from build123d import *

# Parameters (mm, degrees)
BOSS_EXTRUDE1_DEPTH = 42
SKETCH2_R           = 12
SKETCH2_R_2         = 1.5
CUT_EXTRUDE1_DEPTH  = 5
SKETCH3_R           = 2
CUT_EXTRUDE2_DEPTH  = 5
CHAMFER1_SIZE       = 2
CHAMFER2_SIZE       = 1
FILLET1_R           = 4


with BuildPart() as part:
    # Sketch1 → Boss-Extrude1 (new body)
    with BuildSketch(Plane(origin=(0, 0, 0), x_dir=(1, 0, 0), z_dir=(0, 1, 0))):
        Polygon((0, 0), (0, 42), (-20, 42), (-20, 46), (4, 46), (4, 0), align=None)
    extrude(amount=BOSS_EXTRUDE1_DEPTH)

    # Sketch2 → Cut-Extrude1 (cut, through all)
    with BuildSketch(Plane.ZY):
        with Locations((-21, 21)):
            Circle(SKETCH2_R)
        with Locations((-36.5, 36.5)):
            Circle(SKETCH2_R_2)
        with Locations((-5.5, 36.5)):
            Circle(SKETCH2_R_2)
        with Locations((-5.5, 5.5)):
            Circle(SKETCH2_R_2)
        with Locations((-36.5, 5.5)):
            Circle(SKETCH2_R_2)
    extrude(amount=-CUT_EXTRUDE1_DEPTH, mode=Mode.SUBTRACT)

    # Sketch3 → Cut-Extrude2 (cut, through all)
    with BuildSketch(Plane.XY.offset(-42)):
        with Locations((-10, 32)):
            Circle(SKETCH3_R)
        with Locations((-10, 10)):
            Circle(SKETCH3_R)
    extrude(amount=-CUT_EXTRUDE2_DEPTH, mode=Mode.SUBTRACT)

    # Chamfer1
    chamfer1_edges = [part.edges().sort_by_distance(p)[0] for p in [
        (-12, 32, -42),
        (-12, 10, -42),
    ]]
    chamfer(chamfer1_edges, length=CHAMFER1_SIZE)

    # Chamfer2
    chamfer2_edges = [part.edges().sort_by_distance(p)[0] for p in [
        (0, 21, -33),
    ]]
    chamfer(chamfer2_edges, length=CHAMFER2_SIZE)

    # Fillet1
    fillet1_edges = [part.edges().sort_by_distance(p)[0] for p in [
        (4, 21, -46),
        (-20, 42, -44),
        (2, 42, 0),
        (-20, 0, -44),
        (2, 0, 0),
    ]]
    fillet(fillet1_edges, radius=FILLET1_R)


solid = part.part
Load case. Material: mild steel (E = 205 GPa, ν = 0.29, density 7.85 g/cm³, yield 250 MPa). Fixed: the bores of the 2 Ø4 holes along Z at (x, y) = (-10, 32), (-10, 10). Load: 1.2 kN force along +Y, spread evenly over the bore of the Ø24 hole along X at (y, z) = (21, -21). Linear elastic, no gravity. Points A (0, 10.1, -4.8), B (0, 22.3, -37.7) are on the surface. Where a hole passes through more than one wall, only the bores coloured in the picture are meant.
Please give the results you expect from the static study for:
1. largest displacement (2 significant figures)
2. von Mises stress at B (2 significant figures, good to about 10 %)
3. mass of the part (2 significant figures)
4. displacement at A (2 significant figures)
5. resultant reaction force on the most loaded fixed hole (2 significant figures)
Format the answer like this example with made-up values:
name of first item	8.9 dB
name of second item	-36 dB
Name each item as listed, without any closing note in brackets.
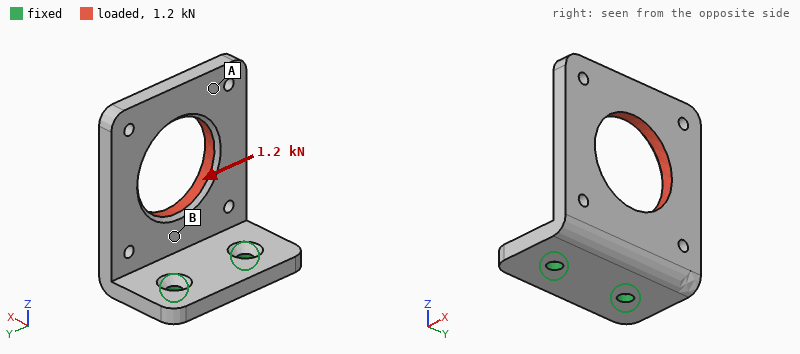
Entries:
largest displacement	0.11 mm
von Mises stress at B	95 MPa
mass of the part	69 g
displacement at A	0.094 mm
resultant reaction force on the most loaded fixed hole	1.4 kN
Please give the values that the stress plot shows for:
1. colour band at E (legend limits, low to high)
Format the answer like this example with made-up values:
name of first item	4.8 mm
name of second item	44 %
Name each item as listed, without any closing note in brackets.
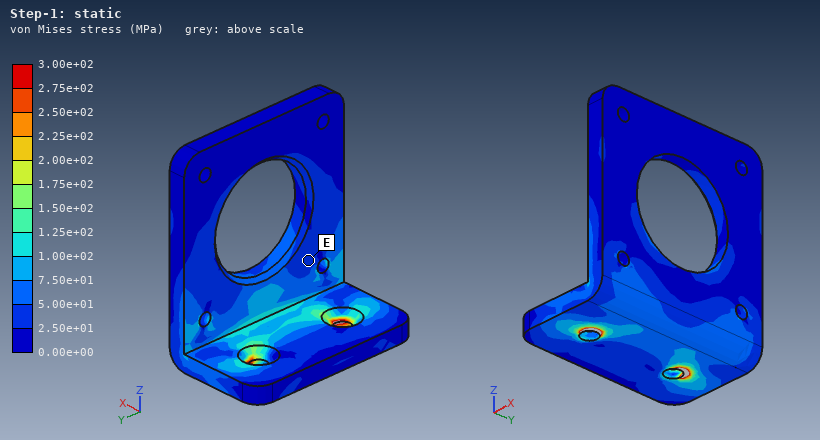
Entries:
colour band at E	2.50e+01 to 5.00e+01 MPa
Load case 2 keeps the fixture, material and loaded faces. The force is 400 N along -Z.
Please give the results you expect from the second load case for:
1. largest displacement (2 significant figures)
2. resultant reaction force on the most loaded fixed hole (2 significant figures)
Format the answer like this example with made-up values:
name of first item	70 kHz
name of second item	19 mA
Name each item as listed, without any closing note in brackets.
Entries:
largest displacement	58 µm
resultant reaction force on the most loaded fixed hole	200 N
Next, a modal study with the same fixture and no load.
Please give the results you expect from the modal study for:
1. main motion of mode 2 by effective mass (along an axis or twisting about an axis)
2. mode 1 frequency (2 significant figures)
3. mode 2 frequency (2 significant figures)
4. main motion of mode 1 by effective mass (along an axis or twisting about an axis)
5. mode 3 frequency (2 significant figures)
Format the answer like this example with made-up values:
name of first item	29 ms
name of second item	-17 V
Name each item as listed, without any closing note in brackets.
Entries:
main motion of mode 2 by effective mass	along Y
mode 1 frequency	1100 Hz
mode 2 frequency	2700 Hz
main motion of mode 1 by effective mass	along X
mode 3 frequency	3700 Hz
